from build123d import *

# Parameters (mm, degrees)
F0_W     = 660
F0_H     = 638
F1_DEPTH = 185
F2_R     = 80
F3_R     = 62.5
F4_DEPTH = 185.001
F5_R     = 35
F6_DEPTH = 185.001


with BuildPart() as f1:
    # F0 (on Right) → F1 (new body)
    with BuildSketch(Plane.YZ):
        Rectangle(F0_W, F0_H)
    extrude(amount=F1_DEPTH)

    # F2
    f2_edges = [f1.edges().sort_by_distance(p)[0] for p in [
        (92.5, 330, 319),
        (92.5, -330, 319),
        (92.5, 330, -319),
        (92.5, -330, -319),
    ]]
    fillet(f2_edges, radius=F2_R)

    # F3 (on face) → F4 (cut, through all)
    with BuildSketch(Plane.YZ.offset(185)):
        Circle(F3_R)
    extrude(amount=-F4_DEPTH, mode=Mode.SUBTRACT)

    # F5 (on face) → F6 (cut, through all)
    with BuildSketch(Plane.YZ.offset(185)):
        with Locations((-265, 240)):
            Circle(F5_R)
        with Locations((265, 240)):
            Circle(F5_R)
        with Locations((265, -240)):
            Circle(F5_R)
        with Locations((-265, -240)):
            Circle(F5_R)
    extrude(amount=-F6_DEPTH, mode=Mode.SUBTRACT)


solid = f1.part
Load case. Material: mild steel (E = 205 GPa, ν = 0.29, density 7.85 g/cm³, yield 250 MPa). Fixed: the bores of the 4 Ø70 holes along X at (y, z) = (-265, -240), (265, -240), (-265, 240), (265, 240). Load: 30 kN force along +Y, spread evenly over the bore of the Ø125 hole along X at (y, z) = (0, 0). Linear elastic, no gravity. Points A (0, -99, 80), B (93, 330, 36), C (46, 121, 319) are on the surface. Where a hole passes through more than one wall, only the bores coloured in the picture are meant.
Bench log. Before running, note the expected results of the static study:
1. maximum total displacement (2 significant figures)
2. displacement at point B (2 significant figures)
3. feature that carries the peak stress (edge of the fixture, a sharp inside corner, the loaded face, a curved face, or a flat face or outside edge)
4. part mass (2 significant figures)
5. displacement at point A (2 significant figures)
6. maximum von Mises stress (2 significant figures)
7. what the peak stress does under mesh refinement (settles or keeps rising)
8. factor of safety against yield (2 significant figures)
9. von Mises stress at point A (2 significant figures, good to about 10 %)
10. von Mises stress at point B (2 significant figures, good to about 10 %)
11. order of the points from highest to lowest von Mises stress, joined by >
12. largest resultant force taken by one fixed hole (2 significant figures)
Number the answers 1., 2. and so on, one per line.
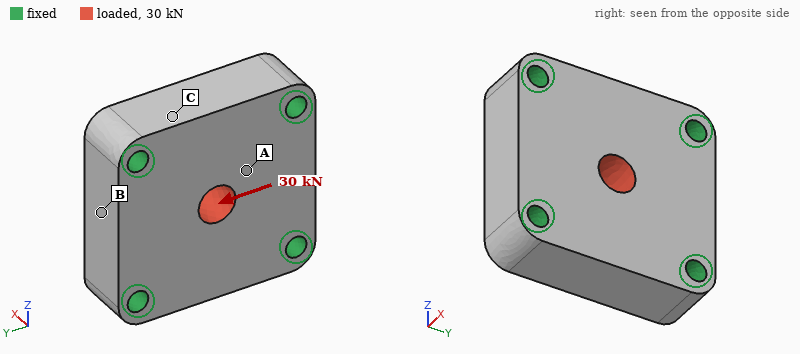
1. 0.52 µm
2. 0.29 µm
3. the loaded face
4. 560 kg
5. 0.35 µm
6. 0.73 MPa
7. settles
8. 340
9. 0.31 MPa
10. 0.17 MPa
11. A > B > C
12. 8.3 kN
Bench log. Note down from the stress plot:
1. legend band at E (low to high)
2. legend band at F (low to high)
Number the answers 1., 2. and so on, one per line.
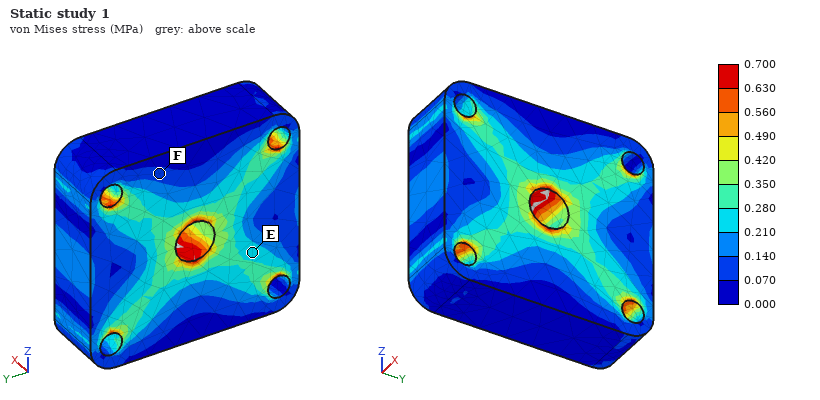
1. 0.210 to 0.280 MPa
2. 0.070 to 0.140 MPa
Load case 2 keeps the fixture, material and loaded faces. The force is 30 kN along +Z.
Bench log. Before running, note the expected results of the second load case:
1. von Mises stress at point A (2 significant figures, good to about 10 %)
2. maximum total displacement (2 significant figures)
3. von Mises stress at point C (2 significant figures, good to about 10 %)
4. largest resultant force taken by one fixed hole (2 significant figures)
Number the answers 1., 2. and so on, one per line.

1. 0.31 MPa
2. 0.58 µm
3. 0.11 MPa
4. 8.5 kN
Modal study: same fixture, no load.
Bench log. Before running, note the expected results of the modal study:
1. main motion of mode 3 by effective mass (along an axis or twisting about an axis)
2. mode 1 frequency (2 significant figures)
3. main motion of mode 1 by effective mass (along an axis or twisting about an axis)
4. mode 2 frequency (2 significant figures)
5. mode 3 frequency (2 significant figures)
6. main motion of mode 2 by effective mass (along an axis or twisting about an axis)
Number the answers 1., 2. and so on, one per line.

1. along Z
2. 1800 Hz
3. along X
4. 2400 Hz
5. 2600 Hz
6. twisting about Y
